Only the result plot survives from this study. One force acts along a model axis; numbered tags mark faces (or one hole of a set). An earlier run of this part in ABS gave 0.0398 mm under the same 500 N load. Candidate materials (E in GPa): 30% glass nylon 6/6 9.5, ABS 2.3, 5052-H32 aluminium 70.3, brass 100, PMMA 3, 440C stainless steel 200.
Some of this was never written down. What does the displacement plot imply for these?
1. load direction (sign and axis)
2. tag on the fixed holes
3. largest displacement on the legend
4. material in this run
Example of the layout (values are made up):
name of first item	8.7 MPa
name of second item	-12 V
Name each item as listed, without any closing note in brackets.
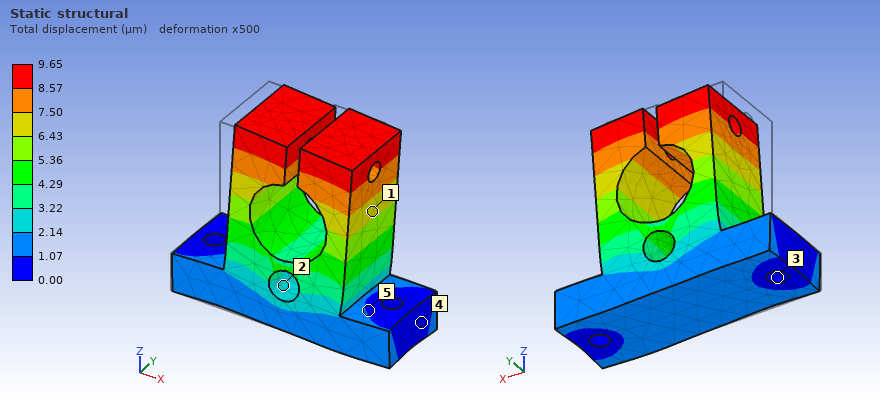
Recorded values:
load direction	+X
tag on the fixed holes	3
largest displacement on the legend	9.65 µm
material in this run	30% glass nylon 6/6
